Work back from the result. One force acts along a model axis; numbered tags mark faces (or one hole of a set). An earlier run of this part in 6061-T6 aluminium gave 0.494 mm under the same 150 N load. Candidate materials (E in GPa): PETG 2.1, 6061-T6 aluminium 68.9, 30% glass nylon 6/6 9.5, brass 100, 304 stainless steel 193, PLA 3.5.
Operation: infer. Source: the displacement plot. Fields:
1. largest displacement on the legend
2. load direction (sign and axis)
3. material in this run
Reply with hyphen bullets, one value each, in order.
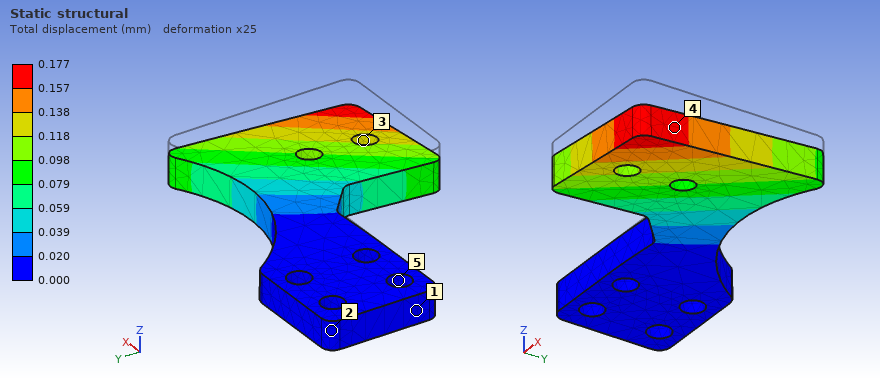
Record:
- 0.177 mm
- -Z
- 304 stainless steel
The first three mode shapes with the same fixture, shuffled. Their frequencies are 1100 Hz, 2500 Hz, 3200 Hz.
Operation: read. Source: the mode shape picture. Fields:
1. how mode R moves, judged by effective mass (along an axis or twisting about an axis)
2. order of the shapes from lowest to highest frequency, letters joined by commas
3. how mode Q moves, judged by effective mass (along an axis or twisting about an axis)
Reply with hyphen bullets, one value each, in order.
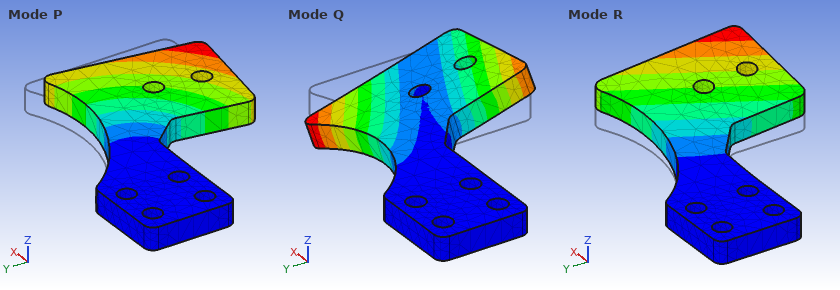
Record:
- along Z
- R, P, Q
- twisting about X
